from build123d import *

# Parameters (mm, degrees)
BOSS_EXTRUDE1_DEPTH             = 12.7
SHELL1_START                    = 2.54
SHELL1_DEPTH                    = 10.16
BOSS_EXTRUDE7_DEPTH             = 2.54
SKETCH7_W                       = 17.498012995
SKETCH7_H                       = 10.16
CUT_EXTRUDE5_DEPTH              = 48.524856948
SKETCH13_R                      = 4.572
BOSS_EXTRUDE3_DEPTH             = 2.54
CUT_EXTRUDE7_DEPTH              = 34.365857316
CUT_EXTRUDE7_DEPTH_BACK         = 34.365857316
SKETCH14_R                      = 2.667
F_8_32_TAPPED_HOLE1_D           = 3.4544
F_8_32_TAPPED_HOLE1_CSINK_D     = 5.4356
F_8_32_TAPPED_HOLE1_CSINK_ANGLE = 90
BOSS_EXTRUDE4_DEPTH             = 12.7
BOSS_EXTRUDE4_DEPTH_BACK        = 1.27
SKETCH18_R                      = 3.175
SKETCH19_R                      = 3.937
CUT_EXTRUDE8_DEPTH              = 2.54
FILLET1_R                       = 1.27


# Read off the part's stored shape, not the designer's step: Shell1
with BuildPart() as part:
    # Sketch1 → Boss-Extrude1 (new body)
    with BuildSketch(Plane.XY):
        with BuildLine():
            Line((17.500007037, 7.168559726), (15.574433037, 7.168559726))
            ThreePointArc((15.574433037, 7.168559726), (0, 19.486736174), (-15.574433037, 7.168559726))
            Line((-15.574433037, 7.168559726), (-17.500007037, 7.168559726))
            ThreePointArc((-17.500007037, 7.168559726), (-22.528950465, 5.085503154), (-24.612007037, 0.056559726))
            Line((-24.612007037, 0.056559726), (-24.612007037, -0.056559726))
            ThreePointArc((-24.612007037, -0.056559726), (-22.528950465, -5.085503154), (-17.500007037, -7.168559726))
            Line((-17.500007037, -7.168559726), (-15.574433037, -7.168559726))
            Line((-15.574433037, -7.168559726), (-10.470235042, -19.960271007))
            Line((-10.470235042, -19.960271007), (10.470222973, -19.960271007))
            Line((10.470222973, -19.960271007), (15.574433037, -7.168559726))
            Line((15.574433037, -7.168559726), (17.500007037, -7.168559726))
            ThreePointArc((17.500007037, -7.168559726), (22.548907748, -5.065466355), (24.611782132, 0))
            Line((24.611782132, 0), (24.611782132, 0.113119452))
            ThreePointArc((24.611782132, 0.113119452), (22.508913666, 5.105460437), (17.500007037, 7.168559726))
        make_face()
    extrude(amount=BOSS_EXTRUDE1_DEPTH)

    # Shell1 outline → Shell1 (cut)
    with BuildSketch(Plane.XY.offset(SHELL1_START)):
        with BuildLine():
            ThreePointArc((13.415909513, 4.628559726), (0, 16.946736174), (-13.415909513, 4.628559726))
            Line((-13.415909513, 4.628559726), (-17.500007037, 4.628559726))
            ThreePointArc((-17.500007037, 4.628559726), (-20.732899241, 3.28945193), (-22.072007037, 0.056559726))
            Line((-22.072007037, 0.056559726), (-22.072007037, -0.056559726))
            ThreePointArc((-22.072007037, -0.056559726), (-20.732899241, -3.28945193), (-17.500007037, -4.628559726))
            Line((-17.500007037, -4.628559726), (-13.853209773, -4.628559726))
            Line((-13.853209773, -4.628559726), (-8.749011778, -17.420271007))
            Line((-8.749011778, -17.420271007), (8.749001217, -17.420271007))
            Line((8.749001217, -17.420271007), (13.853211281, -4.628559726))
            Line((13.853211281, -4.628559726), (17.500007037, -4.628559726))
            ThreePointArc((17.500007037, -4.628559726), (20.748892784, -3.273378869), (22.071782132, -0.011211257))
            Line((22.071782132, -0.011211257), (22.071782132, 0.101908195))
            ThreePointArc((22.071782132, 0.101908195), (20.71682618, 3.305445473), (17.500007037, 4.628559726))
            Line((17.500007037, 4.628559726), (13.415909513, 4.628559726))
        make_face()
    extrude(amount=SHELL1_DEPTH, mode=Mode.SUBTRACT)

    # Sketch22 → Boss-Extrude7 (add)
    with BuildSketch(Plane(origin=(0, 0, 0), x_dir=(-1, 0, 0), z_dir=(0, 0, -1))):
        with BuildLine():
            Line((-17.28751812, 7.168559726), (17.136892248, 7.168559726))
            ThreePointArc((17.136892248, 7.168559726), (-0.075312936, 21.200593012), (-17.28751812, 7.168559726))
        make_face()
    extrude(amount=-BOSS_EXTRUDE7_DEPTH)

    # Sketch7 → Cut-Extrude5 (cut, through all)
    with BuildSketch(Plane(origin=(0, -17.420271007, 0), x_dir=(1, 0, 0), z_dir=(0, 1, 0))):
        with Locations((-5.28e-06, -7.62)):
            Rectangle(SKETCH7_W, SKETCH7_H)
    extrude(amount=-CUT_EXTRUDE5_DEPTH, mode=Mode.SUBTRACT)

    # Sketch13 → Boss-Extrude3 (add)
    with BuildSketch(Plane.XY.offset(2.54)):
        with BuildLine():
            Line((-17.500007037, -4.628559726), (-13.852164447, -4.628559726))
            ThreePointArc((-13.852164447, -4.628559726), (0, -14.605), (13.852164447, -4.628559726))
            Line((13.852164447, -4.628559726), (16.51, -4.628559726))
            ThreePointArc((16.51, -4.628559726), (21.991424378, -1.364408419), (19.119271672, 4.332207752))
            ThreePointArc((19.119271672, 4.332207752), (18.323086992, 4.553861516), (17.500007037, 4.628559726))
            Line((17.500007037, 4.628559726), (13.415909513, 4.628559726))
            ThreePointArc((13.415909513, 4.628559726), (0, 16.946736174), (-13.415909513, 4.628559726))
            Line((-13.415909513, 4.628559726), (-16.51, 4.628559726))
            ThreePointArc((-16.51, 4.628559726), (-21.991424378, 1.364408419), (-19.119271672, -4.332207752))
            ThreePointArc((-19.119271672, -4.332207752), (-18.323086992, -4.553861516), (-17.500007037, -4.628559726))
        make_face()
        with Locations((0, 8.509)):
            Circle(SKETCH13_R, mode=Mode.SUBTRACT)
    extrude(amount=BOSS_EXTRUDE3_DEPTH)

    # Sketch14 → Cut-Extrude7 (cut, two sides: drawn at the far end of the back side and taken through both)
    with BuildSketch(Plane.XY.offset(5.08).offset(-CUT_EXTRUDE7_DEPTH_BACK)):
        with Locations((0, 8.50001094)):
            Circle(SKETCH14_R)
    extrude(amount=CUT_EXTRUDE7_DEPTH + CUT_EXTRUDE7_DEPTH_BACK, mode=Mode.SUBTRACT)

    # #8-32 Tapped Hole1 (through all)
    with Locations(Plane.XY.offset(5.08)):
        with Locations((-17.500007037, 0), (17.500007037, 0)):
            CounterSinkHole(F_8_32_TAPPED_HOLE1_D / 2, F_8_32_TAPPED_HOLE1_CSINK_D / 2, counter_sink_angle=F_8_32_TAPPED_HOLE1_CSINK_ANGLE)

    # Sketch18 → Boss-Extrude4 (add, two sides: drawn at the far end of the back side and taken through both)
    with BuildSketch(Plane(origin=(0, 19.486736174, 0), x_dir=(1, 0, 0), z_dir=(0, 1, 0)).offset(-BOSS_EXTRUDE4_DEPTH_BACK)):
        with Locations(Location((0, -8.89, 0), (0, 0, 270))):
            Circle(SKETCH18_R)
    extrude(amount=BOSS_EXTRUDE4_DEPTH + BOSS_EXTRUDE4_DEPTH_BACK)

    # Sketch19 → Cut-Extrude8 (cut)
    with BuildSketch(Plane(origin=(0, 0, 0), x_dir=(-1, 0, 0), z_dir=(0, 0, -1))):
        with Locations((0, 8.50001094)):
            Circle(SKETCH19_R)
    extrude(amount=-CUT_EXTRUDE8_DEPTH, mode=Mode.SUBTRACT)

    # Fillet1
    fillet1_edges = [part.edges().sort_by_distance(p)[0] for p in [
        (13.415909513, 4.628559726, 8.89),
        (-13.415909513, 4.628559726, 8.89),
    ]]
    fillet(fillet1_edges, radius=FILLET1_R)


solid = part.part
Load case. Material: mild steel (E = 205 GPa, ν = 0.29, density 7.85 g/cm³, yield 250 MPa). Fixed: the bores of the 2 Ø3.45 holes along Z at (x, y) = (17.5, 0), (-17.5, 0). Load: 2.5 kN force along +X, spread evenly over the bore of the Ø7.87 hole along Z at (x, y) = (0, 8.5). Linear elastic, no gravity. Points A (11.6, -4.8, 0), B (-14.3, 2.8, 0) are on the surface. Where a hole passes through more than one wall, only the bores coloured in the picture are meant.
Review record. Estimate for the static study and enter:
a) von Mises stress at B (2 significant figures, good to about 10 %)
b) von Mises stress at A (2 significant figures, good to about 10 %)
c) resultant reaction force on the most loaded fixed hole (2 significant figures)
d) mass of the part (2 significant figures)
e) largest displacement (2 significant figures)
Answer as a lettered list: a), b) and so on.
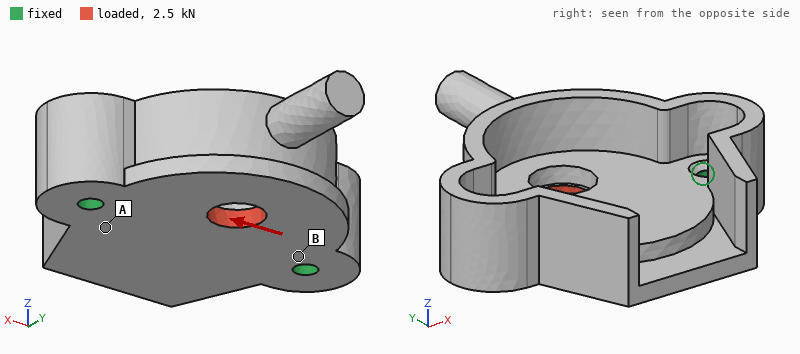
a) 30 MPa
b) 8.8 MPa
c) 1.4 kN
d) 68 g
e) 3.8 µm
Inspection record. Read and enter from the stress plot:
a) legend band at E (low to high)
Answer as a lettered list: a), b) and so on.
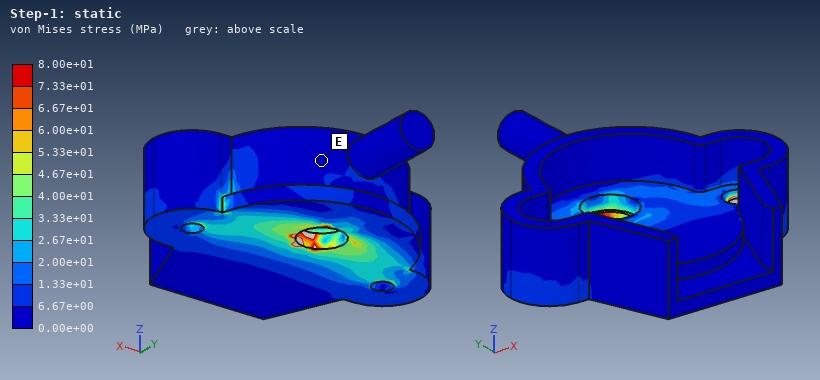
a) 0.00e+00 to 6.67e+00 MPa
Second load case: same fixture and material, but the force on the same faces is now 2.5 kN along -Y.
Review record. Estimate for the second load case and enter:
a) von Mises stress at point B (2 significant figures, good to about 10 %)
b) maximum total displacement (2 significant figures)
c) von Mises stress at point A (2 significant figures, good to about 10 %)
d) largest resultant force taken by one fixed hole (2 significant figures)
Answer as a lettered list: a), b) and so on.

a) 44 MPa
b) 14 µm
c) 18 MPa
d) 1.3 kN
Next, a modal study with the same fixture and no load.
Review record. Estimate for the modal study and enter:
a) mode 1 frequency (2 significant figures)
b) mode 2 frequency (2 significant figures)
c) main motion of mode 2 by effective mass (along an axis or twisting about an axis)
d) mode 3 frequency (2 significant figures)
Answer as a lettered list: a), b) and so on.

a) 5600 Hz
b) 9200 Hz
c) along Z
d) 13 kHz
